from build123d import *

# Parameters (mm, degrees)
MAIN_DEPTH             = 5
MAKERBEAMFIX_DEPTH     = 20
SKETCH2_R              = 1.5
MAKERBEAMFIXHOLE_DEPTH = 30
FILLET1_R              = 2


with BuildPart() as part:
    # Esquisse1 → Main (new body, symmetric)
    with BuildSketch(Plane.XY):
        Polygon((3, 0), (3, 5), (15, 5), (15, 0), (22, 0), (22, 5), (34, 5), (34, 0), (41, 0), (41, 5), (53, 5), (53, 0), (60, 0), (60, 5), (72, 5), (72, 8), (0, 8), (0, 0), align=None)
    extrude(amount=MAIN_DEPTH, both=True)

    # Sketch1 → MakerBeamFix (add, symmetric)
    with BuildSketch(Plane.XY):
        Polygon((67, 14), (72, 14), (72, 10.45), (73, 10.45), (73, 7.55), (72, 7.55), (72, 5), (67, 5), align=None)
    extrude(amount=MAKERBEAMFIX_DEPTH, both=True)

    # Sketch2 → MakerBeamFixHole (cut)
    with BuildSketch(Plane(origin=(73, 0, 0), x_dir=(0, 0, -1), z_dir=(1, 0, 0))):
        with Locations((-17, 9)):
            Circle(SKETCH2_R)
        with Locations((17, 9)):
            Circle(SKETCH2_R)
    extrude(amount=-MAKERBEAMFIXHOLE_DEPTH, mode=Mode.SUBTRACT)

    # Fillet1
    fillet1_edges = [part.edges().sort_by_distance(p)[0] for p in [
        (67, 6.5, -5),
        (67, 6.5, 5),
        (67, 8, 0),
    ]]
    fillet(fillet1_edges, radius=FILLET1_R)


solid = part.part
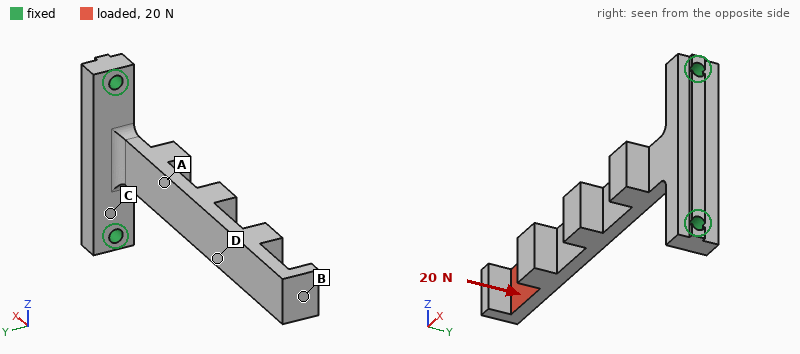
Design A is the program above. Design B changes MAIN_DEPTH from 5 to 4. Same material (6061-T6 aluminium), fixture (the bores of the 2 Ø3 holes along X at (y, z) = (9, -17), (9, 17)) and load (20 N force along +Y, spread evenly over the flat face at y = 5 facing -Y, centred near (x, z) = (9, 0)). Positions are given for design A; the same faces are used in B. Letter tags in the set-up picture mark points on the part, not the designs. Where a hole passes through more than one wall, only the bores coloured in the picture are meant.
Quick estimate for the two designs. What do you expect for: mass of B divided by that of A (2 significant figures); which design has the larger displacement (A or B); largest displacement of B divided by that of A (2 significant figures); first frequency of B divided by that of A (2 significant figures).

0.87
B
1.2
1.0
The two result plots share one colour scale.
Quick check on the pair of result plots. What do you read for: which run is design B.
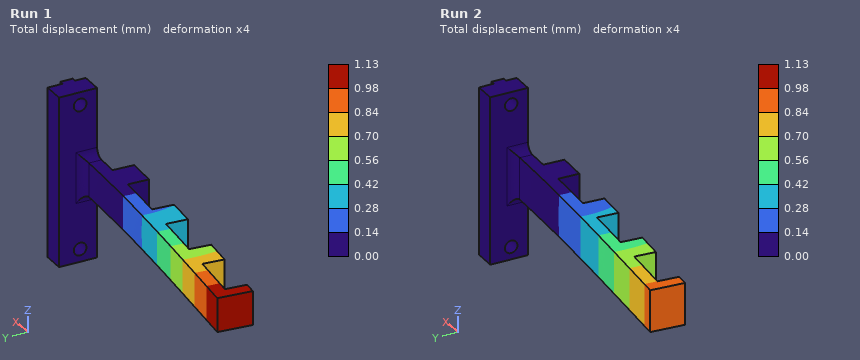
Run 1
